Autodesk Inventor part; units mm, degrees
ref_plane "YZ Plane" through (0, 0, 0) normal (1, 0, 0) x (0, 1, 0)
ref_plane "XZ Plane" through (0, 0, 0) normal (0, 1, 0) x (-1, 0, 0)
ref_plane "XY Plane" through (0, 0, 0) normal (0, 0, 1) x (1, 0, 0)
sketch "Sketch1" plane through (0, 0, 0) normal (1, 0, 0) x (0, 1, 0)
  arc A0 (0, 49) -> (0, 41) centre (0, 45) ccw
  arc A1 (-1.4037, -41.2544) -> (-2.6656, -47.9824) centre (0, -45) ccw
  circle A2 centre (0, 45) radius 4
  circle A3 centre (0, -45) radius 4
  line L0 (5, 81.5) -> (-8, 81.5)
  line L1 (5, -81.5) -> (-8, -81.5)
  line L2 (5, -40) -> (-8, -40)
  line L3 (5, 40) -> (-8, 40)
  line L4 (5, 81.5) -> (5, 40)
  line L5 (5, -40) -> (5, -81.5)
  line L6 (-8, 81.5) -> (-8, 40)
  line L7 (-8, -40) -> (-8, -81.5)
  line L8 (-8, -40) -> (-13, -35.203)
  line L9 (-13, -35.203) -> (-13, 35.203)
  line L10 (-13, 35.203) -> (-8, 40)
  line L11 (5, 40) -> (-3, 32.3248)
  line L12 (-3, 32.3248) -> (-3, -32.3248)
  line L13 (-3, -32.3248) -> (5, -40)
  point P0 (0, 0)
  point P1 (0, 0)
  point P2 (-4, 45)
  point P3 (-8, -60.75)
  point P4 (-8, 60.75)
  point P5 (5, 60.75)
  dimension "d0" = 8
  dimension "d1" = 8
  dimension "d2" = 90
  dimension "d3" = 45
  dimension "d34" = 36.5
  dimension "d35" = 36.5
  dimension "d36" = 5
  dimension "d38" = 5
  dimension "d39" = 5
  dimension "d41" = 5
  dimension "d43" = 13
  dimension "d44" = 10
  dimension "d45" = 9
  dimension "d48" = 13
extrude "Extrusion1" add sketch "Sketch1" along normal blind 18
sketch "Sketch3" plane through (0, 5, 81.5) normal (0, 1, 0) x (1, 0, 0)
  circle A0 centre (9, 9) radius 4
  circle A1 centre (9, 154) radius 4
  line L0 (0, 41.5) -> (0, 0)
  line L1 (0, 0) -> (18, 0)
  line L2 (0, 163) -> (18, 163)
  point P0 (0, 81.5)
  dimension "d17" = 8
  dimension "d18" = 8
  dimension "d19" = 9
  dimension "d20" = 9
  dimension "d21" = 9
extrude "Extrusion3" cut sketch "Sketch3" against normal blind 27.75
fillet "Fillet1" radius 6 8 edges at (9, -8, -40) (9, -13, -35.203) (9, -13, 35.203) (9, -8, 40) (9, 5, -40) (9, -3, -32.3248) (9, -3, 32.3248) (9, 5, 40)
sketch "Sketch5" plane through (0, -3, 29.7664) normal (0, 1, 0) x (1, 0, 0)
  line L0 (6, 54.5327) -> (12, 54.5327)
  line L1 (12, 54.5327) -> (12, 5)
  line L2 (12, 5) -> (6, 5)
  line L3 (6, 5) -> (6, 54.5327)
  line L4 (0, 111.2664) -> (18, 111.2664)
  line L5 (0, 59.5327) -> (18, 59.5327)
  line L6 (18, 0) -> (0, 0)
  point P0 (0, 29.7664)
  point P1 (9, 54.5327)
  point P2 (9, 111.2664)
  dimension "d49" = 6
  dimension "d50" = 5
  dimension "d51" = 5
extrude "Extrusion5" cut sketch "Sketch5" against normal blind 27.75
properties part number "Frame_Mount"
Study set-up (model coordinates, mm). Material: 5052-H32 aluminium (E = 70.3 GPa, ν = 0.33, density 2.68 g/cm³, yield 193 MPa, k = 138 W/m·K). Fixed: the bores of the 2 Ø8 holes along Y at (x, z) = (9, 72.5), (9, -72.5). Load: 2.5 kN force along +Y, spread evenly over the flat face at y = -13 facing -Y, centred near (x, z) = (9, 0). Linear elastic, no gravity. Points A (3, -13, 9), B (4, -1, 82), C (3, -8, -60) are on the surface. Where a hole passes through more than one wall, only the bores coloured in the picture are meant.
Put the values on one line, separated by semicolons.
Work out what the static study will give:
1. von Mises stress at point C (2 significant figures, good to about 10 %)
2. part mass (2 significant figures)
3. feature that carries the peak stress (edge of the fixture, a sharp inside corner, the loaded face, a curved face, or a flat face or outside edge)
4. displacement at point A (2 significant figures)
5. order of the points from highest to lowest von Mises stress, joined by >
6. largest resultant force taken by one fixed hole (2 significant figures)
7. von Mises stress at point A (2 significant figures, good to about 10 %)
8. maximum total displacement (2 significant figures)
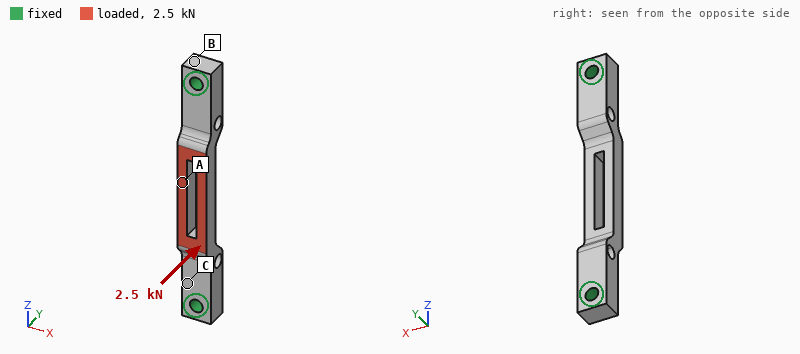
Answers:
31 MPa; 76 g; a curved face; 0.17 mm; A > C > B; 2.9 kN; 83 MPa; 0.18 mm
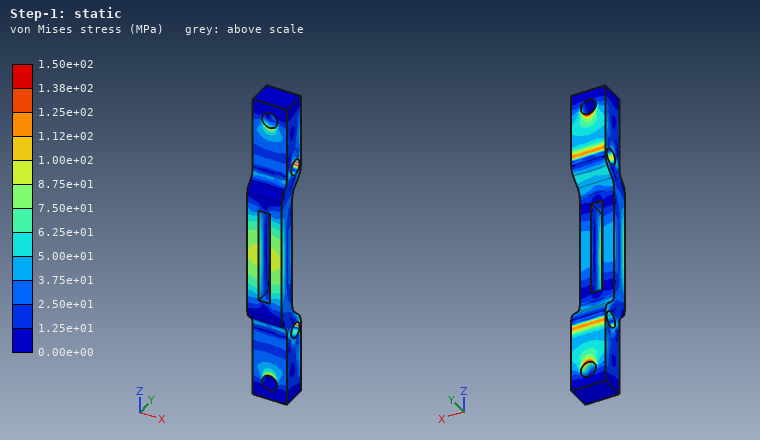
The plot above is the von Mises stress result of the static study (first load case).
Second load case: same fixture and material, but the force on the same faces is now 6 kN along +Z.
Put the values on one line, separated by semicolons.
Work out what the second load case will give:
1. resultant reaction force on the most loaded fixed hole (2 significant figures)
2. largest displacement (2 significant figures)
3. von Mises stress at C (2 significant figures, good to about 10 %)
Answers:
3.0 kN; 19 µm; 18 MPa
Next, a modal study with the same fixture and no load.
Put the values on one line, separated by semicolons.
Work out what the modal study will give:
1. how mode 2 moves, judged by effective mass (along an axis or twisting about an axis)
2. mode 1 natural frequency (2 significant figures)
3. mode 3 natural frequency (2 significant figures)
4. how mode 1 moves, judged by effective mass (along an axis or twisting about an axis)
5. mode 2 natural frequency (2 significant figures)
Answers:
along X; 3900 Hz; 6300 Hz; along Y; 4300 Hz
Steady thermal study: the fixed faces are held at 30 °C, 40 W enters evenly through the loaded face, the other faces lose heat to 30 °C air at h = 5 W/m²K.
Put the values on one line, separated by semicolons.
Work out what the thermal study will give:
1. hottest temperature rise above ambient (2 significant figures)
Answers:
48 K
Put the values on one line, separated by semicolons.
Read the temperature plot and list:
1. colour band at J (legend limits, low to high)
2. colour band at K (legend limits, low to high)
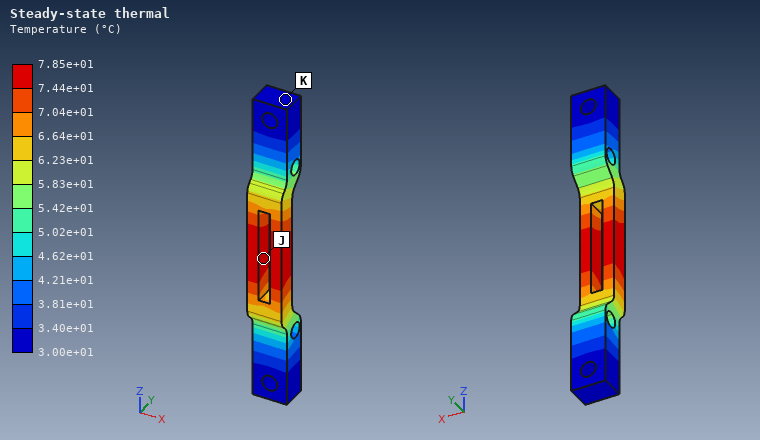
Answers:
7.44e+01 to 7.85e+01 °C; 3.00e+01 to 3.40e+01 °C
